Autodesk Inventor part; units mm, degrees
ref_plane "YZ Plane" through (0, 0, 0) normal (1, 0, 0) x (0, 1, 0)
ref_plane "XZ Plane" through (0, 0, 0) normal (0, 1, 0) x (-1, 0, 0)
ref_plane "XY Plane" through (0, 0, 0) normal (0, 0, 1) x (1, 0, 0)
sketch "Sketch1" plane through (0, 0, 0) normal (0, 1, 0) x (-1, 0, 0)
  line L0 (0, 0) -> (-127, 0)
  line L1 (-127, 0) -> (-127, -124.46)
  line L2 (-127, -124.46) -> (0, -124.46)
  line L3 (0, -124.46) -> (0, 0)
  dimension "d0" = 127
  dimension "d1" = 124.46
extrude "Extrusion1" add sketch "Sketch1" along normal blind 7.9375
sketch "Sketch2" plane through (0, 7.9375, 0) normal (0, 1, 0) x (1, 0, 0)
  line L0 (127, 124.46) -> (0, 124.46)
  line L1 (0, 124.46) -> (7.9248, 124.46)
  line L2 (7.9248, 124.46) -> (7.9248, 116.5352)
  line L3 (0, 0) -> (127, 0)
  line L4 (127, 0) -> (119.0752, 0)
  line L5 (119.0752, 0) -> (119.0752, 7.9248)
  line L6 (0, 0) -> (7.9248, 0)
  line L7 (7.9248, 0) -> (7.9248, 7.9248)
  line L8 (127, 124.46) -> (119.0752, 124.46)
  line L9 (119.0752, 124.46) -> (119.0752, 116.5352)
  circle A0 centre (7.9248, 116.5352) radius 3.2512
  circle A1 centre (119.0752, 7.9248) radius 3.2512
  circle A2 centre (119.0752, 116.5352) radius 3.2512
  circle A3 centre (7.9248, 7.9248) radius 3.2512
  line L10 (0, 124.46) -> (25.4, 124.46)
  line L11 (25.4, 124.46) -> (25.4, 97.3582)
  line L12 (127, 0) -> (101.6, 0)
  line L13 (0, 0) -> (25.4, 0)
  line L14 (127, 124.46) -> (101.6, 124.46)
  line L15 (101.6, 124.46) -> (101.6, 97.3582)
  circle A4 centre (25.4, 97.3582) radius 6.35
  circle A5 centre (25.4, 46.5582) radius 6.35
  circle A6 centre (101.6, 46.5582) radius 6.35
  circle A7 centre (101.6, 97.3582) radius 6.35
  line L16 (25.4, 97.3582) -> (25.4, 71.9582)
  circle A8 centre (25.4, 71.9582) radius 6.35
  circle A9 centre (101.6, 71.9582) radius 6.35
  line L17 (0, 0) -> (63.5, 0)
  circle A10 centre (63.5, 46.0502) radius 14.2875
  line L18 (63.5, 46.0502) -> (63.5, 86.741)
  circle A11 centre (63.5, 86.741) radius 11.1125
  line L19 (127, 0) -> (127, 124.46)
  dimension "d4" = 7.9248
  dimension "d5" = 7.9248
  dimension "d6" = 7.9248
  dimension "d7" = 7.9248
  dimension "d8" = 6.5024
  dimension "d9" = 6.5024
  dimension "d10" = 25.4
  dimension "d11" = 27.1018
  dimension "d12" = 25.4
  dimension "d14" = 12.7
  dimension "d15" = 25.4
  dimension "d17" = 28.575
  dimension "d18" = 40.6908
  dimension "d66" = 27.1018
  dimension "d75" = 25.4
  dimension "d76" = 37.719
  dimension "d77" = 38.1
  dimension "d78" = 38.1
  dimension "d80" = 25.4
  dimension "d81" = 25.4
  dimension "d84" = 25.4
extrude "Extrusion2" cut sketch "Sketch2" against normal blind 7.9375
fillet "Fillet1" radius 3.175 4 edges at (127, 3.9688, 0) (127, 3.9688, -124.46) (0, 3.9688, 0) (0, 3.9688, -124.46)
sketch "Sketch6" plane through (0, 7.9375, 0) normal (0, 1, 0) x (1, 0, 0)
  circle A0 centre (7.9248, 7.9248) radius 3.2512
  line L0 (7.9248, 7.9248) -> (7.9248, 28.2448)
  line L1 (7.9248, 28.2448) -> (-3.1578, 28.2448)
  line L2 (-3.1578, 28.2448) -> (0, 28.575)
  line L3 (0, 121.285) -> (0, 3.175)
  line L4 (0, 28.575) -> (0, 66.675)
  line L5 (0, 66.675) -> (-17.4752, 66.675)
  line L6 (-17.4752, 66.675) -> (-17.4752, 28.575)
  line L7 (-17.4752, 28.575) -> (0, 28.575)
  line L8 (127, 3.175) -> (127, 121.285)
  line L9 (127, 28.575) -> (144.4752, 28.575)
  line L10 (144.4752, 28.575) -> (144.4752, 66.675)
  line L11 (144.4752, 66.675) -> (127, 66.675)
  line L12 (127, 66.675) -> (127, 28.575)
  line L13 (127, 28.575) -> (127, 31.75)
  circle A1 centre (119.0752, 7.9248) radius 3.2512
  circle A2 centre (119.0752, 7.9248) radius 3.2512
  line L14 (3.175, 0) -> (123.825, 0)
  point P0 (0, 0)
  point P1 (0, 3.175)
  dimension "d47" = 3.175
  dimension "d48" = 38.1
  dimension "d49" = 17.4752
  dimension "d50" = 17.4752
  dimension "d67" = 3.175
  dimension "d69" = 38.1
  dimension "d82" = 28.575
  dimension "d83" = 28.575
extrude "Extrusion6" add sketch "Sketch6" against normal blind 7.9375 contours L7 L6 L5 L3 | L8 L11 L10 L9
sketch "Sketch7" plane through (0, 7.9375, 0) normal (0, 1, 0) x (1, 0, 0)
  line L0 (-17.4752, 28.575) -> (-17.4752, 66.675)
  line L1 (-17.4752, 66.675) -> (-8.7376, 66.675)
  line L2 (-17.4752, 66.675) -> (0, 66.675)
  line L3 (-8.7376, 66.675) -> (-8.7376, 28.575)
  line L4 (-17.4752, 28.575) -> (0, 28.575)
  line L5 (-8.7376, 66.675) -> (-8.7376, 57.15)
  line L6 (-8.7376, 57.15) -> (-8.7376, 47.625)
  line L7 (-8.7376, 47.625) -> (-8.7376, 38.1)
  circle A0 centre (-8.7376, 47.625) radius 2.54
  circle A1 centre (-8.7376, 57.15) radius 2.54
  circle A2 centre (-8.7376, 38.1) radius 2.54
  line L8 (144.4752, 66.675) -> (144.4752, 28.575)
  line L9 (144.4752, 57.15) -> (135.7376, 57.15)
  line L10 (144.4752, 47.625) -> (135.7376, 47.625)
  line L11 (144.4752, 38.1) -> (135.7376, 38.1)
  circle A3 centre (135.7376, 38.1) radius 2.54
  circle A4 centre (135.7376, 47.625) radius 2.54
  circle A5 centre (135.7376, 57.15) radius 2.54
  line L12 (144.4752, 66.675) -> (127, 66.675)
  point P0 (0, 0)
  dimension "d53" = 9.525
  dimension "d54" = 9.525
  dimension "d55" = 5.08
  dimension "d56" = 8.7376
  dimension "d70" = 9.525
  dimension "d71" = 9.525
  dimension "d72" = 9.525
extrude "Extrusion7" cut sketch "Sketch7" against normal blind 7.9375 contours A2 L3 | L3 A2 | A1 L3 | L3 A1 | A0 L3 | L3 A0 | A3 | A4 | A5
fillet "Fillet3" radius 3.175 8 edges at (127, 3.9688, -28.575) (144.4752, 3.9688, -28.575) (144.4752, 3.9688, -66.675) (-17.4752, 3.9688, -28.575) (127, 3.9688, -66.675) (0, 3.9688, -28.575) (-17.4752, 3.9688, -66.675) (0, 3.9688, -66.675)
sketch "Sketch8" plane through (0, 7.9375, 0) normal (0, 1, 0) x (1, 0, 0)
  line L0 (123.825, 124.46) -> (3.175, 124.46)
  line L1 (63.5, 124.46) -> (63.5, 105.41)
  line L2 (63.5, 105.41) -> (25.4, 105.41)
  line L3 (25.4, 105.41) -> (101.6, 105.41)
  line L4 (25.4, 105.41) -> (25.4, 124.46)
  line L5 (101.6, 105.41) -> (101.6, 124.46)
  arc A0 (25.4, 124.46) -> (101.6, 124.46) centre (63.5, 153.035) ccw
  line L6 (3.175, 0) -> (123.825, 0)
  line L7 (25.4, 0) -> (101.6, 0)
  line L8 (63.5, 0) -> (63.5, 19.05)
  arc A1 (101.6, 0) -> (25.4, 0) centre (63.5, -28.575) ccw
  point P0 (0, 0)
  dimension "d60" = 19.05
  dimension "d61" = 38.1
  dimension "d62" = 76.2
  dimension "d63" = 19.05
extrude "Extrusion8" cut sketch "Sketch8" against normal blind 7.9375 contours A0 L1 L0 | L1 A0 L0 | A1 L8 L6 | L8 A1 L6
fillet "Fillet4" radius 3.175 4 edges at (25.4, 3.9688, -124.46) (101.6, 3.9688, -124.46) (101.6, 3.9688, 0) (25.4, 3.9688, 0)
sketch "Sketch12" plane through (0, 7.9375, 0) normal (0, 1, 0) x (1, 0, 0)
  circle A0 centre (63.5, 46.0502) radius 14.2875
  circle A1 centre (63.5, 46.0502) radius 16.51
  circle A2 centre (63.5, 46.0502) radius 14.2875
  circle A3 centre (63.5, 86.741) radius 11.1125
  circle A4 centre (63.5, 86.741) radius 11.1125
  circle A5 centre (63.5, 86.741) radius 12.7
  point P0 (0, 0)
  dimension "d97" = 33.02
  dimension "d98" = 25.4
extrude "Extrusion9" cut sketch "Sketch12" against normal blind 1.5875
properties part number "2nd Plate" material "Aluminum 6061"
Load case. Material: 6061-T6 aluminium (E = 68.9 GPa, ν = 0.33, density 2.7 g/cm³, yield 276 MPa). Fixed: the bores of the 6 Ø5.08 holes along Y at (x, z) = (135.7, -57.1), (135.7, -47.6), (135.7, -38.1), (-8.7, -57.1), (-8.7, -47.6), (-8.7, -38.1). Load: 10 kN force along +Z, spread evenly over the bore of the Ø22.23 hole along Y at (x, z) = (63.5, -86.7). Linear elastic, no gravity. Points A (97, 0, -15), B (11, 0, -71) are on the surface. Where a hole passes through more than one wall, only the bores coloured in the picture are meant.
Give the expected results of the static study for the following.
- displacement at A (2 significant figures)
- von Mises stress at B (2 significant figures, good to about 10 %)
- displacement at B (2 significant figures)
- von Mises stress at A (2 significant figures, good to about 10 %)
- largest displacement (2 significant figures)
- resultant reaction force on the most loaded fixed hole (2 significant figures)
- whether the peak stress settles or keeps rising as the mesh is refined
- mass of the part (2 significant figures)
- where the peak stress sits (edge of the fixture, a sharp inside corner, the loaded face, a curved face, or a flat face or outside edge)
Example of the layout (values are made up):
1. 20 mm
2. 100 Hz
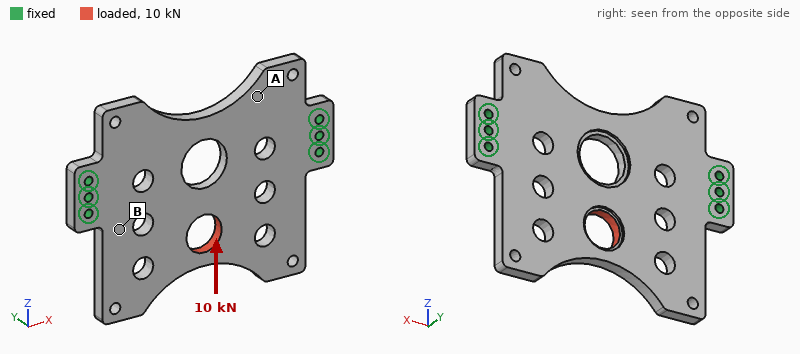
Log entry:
1. 34 µm
2. 31 MPa
3. 22 µm
4. 9.9 MPa
5. 96 µm
6. 3.1 kN
7. keeps rising
8. 280 g
9. edge of the fixture
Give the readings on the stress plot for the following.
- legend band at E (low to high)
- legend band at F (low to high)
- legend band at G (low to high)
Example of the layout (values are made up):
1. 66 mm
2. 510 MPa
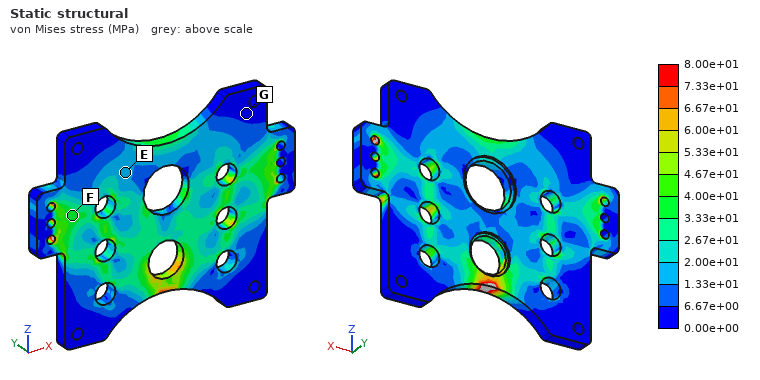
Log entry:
1. 1.33e+01 to 2.00e+01 MPa
2. 3.33e+01 to 4.00e+01 MPa
3. 0.00e+00 to 6.67e+00 MPa
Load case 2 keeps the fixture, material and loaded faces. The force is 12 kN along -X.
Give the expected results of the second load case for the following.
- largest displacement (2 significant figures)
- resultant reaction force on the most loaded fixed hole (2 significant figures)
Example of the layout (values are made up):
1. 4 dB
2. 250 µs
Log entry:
1. 54 µm
2. 3.6 kN
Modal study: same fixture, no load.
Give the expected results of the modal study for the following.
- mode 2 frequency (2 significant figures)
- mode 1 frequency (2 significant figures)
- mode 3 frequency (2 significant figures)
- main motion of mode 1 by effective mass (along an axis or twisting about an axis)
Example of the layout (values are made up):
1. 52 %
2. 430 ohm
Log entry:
1. 1700 Hz
2. 960 Hz
3. 1700 Hz
4. along Y
